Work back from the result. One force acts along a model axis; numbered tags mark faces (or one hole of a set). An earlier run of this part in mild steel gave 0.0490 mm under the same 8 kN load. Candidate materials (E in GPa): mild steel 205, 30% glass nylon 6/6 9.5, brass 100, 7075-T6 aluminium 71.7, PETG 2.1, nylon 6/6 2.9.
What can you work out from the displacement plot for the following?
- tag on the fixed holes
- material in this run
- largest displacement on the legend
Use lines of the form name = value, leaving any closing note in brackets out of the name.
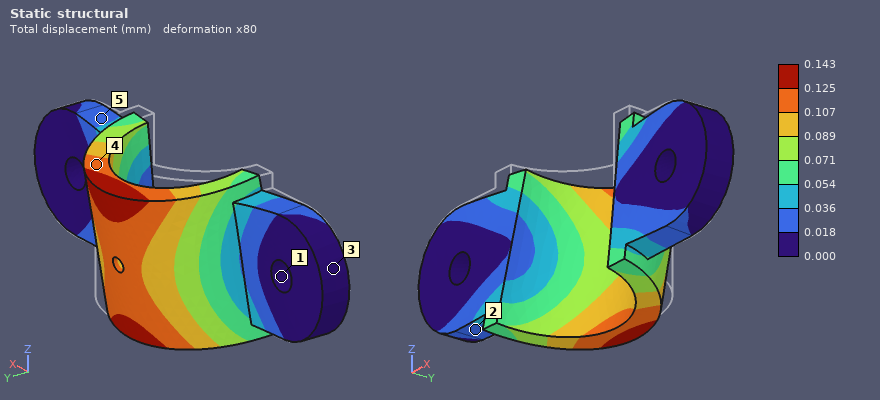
tag on the fixed holes = 1
material in this run = 7075-T6 aluminium
largest displacement on the legend = 0.143 mm
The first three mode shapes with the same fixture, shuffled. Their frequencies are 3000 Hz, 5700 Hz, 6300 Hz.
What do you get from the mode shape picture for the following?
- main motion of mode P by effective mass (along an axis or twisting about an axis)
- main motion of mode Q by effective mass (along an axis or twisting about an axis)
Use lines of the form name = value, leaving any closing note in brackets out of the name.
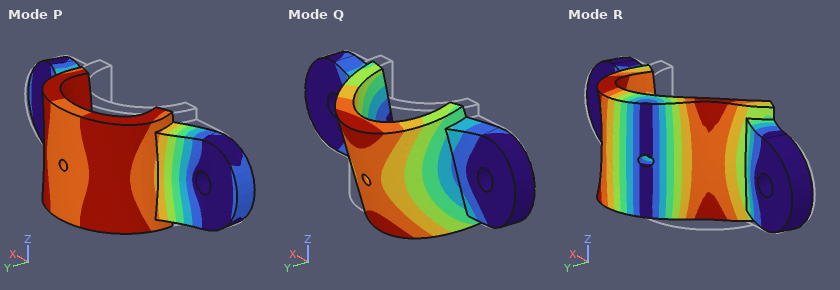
main motion of mode P by effective mass = along Y
main motion of mode Q by effective mass = along Z
